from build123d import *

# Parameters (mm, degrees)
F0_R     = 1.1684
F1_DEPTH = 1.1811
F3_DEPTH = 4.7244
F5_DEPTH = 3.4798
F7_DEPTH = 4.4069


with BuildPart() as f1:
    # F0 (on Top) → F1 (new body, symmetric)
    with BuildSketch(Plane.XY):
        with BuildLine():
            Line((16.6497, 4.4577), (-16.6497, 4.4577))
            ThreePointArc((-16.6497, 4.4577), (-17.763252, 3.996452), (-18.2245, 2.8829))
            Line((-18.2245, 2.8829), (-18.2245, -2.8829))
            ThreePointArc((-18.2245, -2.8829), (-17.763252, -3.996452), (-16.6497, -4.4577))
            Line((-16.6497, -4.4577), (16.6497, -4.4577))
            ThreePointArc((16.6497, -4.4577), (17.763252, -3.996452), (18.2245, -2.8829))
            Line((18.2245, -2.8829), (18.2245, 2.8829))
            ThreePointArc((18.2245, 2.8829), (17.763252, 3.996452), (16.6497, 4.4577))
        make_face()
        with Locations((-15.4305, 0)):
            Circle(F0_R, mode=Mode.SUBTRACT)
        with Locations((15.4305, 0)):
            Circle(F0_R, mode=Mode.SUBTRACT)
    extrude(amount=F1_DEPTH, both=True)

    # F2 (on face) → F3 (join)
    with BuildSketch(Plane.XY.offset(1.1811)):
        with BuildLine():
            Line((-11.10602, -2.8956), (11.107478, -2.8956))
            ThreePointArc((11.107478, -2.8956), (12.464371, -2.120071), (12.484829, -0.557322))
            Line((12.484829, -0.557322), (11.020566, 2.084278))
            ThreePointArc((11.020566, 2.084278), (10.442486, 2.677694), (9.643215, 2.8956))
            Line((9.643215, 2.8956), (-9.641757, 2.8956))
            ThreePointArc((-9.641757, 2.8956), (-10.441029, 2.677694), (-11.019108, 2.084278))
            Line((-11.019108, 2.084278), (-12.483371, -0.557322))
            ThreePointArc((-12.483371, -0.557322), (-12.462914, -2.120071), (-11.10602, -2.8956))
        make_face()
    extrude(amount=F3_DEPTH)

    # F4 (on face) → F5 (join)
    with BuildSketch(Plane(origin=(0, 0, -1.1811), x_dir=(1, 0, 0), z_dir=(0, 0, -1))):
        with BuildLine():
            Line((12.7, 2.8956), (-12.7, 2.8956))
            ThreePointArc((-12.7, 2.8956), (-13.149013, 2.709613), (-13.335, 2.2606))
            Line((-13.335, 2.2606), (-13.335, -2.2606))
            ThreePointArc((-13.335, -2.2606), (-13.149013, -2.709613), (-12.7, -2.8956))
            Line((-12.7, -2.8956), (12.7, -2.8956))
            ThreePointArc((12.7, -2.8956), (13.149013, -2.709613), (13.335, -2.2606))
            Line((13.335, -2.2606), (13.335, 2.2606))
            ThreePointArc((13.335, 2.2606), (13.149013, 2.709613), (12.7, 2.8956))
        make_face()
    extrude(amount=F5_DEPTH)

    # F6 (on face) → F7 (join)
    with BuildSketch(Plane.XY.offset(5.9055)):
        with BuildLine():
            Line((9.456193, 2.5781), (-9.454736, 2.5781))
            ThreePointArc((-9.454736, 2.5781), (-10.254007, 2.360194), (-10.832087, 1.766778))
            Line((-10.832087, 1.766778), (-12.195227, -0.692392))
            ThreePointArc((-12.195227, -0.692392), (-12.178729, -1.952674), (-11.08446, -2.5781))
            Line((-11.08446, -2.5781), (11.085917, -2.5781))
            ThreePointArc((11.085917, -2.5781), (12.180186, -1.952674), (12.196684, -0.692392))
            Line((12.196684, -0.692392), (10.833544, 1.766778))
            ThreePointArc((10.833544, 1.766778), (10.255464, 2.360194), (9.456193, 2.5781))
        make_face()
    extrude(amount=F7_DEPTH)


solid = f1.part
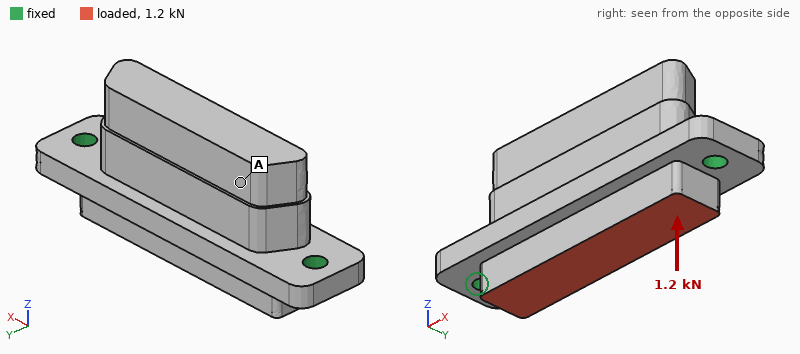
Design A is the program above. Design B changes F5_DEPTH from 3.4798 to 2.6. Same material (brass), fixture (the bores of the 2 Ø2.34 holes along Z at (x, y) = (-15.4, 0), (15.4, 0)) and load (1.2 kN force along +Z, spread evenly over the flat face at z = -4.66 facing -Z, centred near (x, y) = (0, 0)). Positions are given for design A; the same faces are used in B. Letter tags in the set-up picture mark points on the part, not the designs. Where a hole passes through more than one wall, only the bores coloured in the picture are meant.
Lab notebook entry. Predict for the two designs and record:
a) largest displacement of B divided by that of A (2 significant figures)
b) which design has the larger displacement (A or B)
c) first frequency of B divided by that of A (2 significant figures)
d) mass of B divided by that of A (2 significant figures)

1.1
B
1.00
0.94
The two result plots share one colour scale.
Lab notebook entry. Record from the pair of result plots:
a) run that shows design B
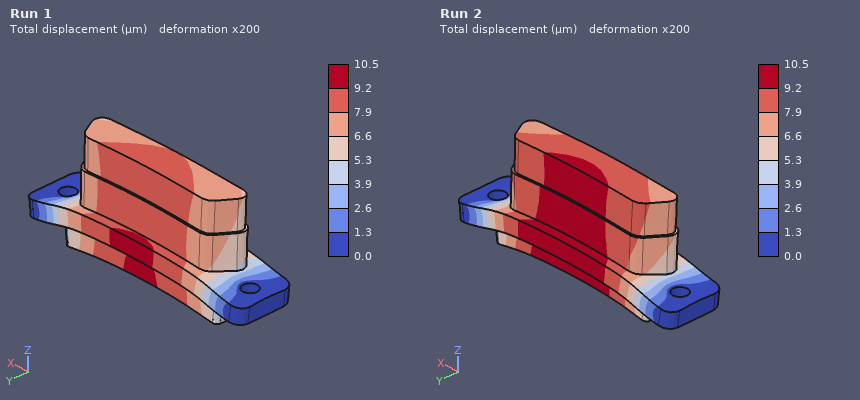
Run 2
